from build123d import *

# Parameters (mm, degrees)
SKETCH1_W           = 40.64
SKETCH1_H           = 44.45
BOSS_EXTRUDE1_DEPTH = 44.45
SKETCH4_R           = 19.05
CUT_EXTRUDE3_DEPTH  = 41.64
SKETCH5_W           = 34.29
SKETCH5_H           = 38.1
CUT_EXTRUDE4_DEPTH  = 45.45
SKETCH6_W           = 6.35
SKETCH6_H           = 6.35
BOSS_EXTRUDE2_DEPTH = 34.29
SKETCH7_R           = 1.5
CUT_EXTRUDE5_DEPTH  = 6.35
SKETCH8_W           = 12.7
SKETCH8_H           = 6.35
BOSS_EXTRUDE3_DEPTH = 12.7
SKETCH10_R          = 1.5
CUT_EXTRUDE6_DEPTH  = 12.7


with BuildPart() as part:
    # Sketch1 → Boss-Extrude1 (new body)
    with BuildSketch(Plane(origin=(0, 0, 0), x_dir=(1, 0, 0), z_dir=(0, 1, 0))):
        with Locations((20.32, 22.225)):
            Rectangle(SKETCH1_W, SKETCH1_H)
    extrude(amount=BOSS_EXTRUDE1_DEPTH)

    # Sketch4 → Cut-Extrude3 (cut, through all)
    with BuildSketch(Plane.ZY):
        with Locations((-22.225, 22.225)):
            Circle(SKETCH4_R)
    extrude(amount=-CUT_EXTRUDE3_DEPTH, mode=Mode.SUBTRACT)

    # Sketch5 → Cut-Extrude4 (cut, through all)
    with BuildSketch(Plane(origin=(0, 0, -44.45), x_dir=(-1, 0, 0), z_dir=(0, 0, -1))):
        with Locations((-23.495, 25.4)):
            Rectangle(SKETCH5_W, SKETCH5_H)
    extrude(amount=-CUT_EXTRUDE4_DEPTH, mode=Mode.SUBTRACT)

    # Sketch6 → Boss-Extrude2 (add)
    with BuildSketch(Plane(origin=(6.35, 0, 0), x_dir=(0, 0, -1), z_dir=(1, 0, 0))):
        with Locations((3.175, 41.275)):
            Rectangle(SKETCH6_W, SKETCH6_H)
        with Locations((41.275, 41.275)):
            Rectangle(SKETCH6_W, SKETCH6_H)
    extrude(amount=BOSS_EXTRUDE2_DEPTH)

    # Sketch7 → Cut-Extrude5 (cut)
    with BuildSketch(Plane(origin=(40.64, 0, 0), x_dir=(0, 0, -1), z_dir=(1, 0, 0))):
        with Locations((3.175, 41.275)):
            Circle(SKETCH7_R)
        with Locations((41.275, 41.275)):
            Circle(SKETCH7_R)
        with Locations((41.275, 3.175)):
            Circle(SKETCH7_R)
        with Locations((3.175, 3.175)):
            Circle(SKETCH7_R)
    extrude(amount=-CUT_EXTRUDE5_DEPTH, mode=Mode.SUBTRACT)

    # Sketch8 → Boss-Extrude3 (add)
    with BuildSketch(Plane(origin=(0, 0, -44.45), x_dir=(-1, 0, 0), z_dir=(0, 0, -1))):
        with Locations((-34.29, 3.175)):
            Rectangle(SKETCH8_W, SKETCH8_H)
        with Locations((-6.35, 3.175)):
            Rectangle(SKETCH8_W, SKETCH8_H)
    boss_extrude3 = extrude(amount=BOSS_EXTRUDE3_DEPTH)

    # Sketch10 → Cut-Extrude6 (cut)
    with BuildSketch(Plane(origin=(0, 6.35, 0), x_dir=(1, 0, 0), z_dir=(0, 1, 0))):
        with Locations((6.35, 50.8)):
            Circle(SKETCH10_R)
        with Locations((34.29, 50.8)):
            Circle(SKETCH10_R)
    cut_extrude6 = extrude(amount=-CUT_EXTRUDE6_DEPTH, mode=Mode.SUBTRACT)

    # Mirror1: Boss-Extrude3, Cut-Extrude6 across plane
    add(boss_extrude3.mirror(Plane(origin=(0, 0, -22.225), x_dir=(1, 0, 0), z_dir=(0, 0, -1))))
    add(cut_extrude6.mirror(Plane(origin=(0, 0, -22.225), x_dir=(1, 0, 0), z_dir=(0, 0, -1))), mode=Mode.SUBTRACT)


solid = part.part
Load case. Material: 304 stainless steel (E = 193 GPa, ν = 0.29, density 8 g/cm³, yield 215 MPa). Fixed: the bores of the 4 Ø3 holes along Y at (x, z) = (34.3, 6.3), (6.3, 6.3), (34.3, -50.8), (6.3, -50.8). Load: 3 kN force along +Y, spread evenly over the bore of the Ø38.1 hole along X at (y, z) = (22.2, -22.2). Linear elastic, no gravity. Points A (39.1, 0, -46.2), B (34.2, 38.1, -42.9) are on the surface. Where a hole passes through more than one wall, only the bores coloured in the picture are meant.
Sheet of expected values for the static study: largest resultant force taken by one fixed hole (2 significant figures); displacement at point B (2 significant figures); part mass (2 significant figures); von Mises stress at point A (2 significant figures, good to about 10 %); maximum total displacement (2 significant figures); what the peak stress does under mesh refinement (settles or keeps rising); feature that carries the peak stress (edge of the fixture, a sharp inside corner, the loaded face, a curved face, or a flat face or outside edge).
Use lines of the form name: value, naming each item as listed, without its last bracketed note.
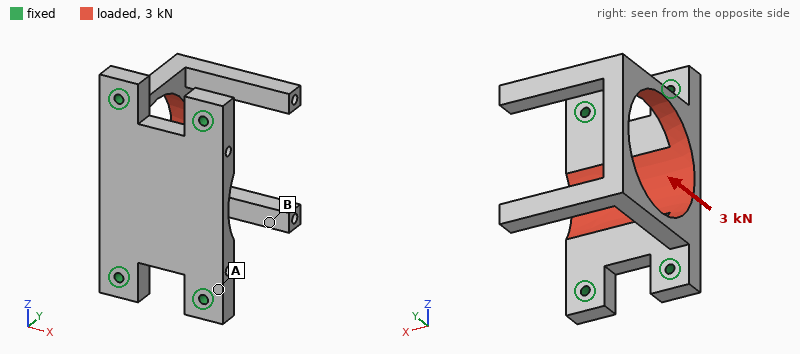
largest resultant force taken by one fixed hole: 1.3 kN
displacement at point B: 7.5 µm
part mass: 160 g
von Mises stress at point A: 40 MPa
maximum total displacement: 25 µm
what the peak stress does under mesh refinement: keeps rising
feature that carries the peak stress: edge of the fixture
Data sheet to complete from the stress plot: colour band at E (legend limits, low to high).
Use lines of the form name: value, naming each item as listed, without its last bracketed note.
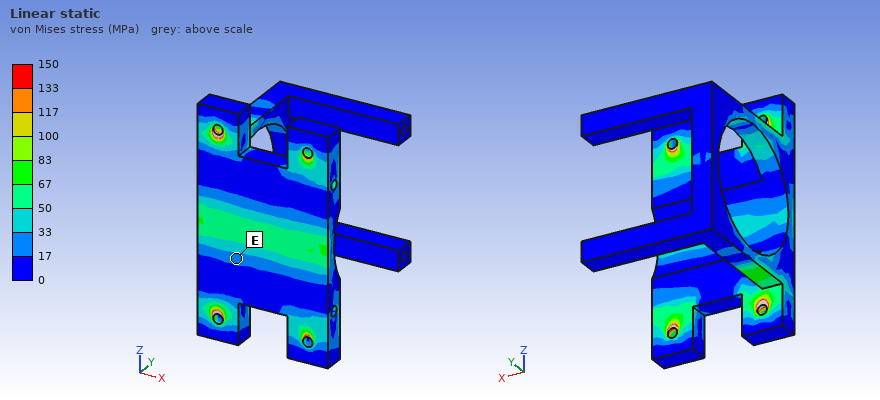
colour band at E: 17 to 33 MPa
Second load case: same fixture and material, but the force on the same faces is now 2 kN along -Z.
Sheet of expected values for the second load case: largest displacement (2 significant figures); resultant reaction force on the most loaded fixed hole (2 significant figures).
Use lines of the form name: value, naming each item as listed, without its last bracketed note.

largest displacement: 54 µm
resultant reaction force on the most loaded fixed hole: 730 N
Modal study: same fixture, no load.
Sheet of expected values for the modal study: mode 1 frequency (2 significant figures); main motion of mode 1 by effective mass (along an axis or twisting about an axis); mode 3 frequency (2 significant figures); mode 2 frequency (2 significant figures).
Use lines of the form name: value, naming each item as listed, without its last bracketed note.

mode 1 frequency: 970 Hz
main motion of mode 1 by effective mass: along X
mode 3 frequency: 2100 Hz
mode 2 frequency: 1300 Hz
